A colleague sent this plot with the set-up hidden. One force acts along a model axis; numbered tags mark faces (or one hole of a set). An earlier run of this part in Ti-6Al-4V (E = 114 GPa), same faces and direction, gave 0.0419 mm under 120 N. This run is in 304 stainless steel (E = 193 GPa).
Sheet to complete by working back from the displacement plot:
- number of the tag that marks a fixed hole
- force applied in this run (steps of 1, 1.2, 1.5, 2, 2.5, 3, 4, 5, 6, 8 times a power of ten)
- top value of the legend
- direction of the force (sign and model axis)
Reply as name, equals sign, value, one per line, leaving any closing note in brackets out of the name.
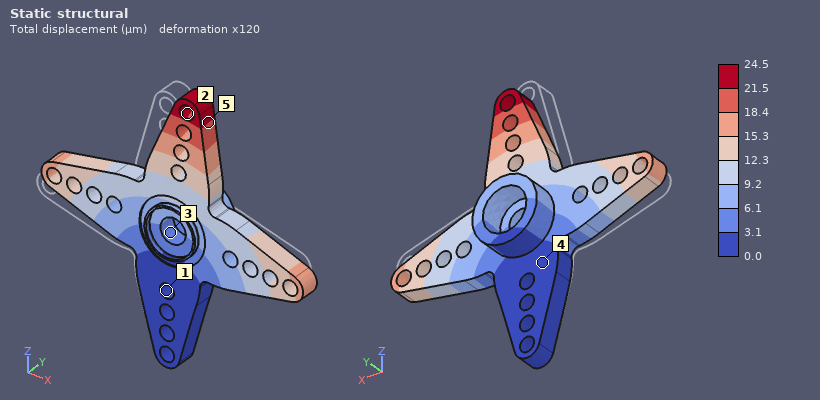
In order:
number of the tag that marks a fixed hole = 1
force applied in this run = 120 N
top value of the legend = 24.5 µm
direction of the force = +X
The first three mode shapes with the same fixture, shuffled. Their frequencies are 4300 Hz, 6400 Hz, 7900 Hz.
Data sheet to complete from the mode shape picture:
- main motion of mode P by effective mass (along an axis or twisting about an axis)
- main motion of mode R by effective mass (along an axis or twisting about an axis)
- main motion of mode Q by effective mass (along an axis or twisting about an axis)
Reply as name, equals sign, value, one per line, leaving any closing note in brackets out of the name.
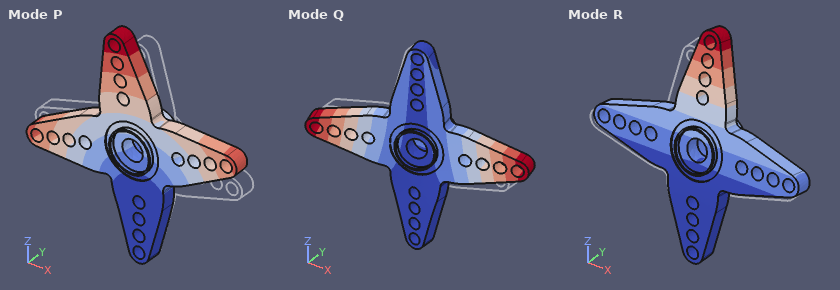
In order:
main motion of mode P by effective mass = along X
main motion of mode R by effective mass = along Y
main motion of mode Q by effective mass = twisting about Z
